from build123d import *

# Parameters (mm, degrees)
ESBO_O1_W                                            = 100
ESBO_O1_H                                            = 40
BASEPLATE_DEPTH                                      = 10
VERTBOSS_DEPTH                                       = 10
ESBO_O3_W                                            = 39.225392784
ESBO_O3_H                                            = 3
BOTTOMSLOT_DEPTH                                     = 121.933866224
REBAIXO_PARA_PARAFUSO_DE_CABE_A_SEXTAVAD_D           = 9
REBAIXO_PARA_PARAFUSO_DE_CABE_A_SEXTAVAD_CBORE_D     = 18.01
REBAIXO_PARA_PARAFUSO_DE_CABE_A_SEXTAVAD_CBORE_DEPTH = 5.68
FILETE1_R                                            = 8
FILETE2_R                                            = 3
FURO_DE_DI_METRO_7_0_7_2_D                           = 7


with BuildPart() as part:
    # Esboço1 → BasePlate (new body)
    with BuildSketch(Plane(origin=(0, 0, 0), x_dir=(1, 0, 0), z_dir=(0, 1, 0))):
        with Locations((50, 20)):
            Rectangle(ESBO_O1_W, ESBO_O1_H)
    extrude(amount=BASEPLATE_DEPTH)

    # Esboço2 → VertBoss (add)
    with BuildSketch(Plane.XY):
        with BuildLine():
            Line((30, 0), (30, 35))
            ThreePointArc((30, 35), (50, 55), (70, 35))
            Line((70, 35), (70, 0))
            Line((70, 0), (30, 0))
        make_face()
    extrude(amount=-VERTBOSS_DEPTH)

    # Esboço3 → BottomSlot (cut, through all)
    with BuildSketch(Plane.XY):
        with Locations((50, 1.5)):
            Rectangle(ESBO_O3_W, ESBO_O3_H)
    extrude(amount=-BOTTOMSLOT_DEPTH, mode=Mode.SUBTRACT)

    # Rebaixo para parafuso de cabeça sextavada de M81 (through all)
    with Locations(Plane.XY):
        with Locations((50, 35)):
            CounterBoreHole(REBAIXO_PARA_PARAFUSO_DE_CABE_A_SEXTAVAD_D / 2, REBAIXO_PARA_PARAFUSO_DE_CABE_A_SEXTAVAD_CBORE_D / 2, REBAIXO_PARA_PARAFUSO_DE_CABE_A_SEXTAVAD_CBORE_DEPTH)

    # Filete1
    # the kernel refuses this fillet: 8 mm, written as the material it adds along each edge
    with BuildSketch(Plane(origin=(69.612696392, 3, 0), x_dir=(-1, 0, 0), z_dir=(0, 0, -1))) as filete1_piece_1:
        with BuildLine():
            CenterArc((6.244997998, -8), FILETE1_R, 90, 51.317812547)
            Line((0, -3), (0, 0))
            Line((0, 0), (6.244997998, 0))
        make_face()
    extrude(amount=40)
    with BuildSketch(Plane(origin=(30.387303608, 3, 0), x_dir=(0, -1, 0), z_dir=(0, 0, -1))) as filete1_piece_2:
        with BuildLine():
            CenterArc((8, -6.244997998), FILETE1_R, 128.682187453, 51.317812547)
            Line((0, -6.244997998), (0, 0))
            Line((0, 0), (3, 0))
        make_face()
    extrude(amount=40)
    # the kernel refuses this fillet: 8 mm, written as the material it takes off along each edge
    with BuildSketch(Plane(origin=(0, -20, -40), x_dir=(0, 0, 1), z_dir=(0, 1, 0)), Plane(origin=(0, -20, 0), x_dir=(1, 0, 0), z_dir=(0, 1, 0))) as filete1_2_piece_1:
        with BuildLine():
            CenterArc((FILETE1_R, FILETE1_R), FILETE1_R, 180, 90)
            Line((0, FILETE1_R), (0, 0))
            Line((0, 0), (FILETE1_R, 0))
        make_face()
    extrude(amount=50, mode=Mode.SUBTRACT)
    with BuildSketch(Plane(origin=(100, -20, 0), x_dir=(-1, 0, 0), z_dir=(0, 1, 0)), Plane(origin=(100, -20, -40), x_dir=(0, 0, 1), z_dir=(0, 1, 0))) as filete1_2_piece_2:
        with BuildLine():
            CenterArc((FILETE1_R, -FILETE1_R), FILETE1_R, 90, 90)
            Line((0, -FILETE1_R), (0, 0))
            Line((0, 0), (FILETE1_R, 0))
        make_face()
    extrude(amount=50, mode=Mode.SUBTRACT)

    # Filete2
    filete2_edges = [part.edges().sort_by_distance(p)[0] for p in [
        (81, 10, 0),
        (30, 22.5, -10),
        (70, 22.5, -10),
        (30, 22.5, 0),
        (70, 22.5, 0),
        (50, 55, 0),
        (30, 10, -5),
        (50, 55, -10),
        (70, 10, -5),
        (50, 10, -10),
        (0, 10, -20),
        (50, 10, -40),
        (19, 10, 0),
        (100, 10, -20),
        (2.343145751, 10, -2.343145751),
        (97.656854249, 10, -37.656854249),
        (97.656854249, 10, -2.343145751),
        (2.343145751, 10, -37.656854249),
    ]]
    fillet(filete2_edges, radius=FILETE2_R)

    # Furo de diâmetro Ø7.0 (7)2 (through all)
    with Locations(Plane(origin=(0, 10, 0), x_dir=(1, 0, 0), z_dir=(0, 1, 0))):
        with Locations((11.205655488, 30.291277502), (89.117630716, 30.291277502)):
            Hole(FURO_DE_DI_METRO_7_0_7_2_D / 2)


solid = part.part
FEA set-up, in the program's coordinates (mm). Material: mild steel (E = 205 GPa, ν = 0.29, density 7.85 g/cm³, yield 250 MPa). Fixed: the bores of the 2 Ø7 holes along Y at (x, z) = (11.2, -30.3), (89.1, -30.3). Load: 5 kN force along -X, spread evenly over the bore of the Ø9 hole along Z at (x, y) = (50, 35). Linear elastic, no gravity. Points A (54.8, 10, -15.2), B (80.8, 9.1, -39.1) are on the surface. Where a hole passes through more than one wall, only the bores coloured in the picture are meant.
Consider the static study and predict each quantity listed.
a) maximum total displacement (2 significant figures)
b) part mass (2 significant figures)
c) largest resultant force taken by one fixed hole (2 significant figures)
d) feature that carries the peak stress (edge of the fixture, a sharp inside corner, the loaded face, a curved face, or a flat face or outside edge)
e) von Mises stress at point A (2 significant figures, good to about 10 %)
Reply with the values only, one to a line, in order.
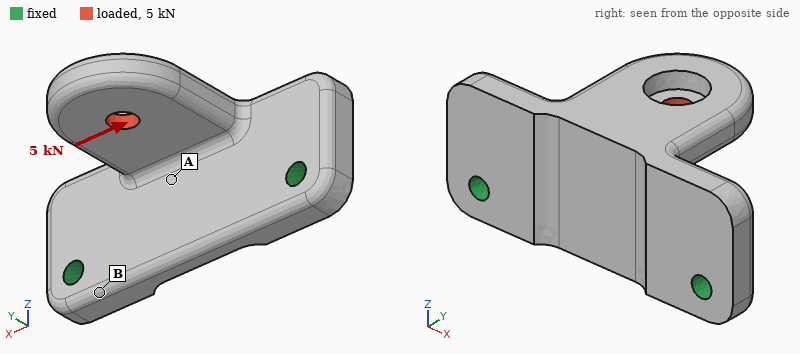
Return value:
74 µm
380 g
3.7 kN
a curved face
65 MPa
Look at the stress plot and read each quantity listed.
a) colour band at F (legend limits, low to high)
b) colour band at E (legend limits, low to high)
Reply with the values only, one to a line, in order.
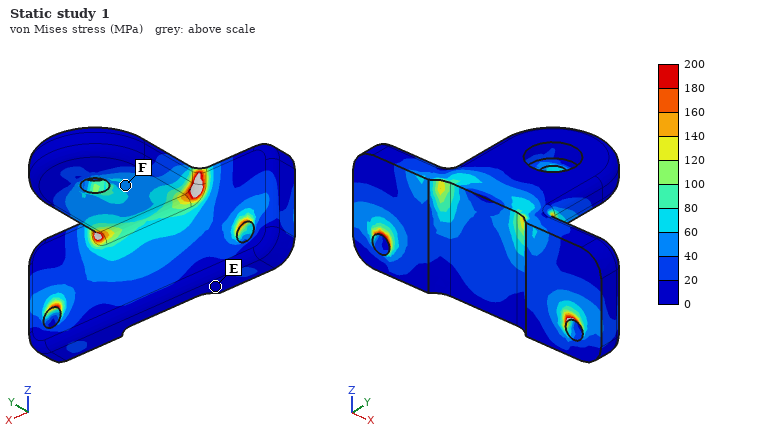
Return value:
40 to 60 MPa
0 to 20 MPa
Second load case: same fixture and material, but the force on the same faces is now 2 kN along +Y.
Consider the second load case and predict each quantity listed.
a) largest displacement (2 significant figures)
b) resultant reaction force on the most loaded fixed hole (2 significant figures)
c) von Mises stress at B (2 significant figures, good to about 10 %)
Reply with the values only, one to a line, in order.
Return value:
32 µm
1.1 kN
16 MPa
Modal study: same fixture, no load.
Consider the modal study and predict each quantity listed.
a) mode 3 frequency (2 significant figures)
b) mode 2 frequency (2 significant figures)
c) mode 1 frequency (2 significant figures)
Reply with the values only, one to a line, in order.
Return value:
4800 Hz
4700 Hz
2300 Hz
